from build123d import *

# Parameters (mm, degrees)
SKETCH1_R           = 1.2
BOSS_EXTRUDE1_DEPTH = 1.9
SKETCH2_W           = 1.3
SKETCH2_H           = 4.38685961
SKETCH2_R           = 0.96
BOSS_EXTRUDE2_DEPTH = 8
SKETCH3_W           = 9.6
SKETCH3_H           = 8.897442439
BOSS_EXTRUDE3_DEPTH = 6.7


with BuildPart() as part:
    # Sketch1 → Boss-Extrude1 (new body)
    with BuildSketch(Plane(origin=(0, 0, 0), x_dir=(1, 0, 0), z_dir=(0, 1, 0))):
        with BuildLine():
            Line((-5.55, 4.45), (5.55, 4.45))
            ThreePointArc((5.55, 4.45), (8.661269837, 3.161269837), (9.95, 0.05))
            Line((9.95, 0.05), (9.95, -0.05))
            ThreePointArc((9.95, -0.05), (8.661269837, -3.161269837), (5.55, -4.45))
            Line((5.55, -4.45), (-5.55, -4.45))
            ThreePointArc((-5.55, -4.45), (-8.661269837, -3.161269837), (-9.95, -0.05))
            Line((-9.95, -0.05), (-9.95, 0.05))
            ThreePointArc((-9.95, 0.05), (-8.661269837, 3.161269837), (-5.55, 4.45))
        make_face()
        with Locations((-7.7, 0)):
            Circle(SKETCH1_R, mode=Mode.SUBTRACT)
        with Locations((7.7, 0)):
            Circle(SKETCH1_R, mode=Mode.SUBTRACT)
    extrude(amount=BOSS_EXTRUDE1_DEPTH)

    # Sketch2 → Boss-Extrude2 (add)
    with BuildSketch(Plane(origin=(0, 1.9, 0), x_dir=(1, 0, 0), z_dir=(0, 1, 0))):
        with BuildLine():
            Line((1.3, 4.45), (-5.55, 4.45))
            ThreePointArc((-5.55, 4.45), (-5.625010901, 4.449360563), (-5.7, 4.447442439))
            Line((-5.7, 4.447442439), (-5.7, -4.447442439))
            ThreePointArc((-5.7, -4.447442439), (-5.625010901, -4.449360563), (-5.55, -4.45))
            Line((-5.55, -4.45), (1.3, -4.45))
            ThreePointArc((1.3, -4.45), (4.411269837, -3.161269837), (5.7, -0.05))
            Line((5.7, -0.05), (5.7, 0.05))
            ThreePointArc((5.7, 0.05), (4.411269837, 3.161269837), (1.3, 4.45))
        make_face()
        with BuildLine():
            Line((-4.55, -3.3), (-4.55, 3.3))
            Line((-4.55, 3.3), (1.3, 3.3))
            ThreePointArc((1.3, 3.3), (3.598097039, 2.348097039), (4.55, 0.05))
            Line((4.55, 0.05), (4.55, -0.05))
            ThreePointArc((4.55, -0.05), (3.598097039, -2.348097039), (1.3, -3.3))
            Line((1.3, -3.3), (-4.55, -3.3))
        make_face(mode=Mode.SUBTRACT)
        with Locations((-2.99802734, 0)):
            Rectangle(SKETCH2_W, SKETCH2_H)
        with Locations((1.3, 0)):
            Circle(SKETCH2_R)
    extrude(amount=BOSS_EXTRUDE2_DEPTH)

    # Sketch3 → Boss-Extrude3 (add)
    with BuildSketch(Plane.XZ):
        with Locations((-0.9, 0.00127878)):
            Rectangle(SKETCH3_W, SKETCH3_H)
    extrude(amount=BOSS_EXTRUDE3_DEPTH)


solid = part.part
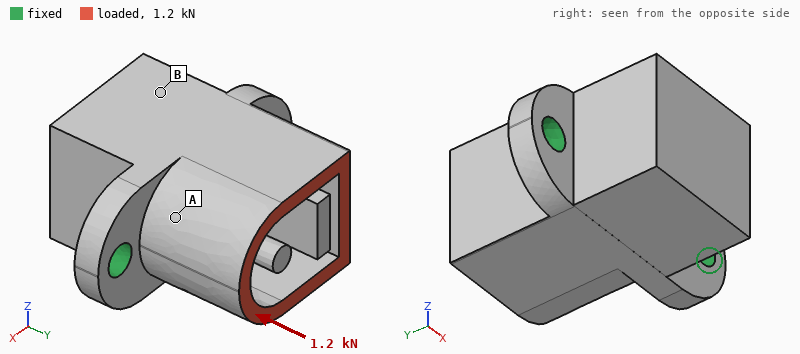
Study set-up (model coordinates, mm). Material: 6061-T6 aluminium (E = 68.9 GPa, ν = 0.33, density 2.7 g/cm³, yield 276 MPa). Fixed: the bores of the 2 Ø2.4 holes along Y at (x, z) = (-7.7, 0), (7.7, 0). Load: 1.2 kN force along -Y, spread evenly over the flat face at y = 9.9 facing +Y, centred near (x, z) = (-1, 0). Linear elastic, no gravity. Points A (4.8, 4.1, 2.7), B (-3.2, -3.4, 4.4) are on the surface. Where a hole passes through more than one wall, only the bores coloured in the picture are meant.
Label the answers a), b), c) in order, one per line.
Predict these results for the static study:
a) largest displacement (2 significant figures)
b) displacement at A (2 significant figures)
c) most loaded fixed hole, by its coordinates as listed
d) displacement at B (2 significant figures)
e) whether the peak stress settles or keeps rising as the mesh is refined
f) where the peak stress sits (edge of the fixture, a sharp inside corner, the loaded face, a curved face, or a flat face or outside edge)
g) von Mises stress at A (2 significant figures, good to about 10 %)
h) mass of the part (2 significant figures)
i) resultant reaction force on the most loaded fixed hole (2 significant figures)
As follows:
a) 15 µm
b) 10.0 µm
c) (-7.7, 0)
d) 8.1 µm
e) keeps rising
f) edge of the fixture
g) 43 MPa
h) 3.3 g
i) 640 N
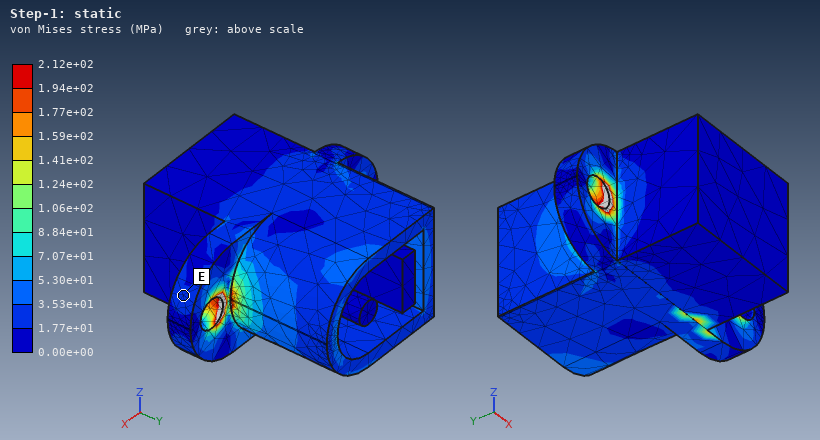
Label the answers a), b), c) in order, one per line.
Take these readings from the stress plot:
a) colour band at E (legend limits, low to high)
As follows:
a) 1.77e+01 to 3.53e+01 MPa
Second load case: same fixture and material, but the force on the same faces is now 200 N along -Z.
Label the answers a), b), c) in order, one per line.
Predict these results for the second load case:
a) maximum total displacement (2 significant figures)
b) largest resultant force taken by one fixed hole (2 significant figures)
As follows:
a) 47 µm
b) 100 N
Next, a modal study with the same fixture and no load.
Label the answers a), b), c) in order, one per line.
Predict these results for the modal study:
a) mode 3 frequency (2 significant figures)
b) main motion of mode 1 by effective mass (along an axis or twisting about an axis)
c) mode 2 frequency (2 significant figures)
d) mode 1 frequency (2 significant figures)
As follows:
a) 19 kHz
b) twisting about X
c) 15 kHz
d) 12 kHz
